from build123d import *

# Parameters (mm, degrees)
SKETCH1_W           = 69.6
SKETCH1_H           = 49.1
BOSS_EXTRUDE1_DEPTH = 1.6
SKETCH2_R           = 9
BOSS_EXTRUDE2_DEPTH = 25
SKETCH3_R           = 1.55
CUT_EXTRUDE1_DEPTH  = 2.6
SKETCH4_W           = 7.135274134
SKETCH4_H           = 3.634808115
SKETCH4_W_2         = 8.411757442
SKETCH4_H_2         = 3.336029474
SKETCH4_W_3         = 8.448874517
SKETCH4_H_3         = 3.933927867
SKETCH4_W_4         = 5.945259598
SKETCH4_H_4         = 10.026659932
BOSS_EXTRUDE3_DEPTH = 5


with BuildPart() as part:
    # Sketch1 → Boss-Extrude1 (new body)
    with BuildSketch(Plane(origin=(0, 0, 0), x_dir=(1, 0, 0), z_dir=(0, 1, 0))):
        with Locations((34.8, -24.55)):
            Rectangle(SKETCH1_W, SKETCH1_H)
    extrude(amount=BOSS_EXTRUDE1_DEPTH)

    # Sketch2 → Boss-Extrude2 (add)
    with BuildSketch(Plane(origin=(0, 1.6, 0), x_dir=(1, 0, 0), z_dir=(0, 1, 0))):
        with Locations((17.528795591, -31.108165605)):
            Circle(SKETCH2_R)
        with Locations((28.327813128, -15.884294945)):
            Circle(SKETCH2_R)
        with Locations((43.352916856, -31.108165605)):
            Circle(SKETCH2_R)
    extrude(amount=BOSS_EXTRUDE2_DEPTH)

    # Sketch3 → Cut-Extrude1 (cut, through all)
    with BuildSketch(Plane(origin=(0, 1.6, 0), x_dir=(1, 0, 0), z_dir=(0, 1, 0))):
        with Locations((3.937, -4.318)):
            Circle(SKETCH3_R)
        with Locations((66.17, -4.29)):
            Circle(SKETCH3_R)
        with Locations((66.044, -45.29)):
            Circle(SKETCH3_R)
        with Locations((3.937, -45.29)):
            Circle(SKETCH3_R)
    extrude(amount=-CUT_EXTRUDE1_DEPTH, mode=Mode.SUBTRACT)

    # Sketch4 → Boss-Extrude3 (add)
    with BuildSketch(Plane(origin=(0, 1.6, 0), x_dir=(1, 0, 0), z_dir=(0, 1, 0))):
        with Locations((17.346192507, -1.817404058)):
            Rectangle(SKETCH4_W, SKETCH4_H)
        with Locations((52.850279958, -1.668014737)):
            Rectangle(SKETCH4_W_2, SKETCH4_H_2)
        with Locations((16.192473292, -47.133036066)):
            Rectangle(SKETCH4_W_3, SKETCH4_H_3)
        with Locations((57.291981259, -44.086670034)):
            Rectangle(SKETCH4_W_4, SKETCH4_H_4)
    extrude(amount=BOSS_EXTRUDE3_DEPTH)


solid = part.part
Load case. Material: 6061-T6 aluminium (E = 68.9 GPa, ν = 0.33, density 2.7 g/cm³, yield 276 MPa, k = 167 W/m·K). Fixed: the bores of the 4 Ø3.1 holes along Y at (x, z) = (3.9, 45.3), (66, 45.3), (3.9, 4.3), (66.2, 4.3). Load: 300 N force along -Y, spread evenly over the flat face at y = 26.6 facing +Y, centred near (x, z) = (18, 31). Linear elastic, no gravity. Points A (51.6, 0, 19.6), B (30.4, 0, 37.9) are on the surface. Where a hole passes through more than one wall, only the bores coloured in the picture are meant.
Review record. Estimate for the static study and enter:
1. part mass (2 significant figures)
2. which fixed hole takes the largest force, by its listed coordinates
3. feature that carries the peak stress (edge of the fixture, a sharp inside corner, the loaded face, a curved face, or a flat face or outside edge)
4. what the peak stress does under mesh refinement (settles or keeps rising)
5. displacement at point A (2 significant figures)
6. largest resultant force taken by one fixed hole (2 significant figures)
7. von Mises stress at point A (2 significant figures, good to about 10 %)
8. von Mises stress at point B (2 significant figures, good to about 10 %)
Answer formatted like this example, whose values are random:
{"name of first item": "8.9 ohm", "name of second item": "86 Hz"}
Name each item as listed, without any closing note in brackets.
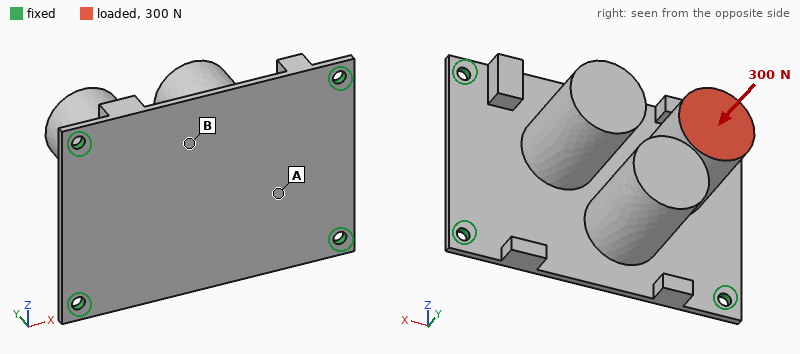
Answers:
{"part mass": "68 g", "which fixed hole takes the largest force, by its listed coordinates": "(3.9, 45.3)", "feature that carries the peak stress": "edge of the fixture", "what the peak stress does under mesh refinement": "keeps rising", "displacement at point A": "0.080 mm", "largest resultant force taken by one fixed hole": "180 N", "von Mises stress at point A": "15 MPa", "von Mises stress at point B": "40 MPa"}
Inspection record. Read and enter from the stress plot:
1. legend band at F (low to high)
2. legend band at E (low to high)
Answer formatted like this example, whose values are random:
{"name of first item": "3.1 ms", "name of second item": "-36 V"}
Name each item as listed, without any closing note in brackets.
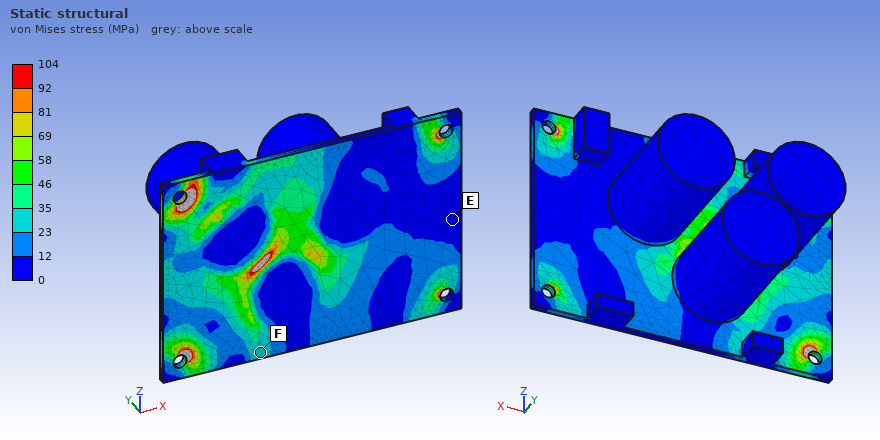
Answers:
{"legend band at F": "23 to 35 MPa", "legend band at E": "0 to 12 MPa"}
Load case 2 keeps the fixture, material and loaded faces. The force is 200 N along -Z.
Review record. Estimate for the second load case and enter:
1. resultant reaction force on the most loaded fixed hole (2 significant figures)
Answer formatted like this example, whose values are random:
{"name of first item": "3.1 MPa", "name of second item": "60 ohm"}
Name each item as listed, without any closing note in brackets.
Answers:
{"resultant reaction force on the most loaded fixed hole": "160 N"}
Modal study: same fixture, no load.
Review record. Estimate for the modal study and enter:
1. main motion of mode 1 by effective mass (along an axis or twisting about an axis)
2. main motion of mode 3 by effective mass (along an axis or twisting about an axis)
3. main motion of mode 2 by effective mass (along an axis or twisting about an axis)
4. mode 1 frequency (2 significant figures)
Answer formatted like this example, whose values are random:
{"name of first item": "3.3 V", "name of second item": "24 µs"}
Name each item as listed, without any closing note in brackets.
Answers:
{"main motion of mode 1 by effective mass": "along Y", "main motion of mode 3 by effective mass": "along X", "main motion of mode 2 by effective mass": "along Z", "mode 1 frequency": "780 Hz"}
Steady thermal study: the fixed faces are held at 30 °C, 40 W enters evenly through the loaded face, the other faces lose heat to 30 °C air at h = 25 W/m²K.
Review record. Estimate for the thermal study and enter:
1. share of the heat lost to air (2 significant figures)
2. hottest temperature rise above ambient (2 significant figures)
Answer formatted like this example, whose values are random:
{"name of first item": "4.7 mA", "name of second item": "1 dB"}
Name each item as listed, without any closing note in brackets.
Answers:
{"share of the heat lost to air": "18 %", "hottest temperature rise above ambient": "66 K"}
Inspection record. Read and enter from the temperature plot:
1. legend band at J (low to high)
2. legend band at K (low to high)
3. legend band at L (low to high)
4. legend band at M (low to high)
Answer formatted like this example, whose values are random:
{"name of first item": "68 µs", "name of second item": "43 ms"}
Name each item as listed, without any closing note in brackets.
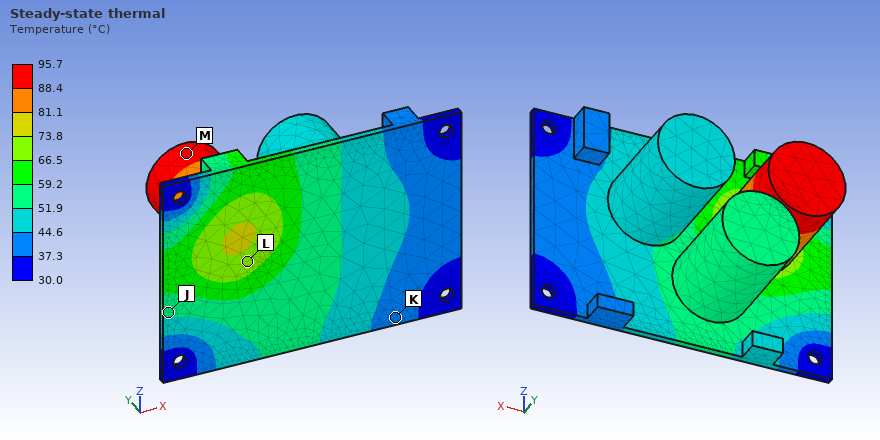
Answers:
{"legend band at J": "51.9 to 59.2 °C", "legend band at K": "37.3 to 44.6 °C", "legend band at L": "66.5 to 73.8 °C", "legend band at M": "88.4 to 95.7 °C"}
